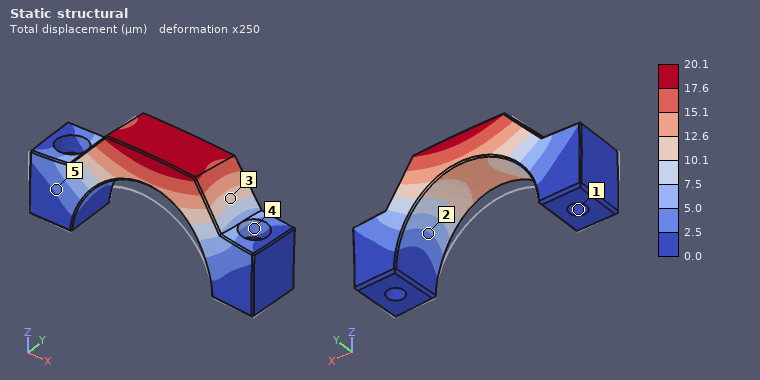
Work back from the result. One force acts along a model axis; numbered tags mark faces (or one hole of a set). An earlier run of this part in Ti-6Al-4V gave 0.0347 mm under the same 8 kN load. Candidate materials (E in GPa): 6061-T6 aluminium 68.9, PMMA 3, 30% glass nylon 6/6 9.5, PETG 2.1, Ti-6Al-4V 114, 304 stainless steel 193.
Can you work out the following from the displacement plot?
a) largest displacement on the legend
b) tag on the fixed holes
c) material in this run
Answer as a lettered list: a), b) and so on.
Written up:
a) 20.1 µm
b) 1
c) 304 stainless steel
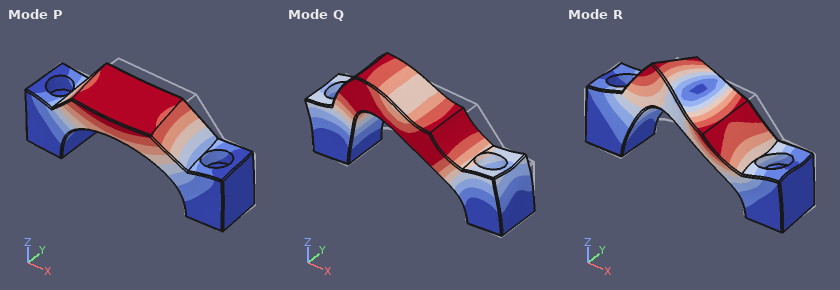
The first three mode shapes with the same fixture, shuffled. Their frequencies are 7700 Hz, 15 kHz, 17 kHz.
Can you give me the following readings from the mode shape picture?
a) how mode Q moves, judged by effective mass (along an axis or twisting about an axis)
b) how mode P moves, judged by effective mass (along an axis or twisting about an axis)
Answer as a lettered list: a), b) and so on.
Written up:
a) along X
b) along Y
